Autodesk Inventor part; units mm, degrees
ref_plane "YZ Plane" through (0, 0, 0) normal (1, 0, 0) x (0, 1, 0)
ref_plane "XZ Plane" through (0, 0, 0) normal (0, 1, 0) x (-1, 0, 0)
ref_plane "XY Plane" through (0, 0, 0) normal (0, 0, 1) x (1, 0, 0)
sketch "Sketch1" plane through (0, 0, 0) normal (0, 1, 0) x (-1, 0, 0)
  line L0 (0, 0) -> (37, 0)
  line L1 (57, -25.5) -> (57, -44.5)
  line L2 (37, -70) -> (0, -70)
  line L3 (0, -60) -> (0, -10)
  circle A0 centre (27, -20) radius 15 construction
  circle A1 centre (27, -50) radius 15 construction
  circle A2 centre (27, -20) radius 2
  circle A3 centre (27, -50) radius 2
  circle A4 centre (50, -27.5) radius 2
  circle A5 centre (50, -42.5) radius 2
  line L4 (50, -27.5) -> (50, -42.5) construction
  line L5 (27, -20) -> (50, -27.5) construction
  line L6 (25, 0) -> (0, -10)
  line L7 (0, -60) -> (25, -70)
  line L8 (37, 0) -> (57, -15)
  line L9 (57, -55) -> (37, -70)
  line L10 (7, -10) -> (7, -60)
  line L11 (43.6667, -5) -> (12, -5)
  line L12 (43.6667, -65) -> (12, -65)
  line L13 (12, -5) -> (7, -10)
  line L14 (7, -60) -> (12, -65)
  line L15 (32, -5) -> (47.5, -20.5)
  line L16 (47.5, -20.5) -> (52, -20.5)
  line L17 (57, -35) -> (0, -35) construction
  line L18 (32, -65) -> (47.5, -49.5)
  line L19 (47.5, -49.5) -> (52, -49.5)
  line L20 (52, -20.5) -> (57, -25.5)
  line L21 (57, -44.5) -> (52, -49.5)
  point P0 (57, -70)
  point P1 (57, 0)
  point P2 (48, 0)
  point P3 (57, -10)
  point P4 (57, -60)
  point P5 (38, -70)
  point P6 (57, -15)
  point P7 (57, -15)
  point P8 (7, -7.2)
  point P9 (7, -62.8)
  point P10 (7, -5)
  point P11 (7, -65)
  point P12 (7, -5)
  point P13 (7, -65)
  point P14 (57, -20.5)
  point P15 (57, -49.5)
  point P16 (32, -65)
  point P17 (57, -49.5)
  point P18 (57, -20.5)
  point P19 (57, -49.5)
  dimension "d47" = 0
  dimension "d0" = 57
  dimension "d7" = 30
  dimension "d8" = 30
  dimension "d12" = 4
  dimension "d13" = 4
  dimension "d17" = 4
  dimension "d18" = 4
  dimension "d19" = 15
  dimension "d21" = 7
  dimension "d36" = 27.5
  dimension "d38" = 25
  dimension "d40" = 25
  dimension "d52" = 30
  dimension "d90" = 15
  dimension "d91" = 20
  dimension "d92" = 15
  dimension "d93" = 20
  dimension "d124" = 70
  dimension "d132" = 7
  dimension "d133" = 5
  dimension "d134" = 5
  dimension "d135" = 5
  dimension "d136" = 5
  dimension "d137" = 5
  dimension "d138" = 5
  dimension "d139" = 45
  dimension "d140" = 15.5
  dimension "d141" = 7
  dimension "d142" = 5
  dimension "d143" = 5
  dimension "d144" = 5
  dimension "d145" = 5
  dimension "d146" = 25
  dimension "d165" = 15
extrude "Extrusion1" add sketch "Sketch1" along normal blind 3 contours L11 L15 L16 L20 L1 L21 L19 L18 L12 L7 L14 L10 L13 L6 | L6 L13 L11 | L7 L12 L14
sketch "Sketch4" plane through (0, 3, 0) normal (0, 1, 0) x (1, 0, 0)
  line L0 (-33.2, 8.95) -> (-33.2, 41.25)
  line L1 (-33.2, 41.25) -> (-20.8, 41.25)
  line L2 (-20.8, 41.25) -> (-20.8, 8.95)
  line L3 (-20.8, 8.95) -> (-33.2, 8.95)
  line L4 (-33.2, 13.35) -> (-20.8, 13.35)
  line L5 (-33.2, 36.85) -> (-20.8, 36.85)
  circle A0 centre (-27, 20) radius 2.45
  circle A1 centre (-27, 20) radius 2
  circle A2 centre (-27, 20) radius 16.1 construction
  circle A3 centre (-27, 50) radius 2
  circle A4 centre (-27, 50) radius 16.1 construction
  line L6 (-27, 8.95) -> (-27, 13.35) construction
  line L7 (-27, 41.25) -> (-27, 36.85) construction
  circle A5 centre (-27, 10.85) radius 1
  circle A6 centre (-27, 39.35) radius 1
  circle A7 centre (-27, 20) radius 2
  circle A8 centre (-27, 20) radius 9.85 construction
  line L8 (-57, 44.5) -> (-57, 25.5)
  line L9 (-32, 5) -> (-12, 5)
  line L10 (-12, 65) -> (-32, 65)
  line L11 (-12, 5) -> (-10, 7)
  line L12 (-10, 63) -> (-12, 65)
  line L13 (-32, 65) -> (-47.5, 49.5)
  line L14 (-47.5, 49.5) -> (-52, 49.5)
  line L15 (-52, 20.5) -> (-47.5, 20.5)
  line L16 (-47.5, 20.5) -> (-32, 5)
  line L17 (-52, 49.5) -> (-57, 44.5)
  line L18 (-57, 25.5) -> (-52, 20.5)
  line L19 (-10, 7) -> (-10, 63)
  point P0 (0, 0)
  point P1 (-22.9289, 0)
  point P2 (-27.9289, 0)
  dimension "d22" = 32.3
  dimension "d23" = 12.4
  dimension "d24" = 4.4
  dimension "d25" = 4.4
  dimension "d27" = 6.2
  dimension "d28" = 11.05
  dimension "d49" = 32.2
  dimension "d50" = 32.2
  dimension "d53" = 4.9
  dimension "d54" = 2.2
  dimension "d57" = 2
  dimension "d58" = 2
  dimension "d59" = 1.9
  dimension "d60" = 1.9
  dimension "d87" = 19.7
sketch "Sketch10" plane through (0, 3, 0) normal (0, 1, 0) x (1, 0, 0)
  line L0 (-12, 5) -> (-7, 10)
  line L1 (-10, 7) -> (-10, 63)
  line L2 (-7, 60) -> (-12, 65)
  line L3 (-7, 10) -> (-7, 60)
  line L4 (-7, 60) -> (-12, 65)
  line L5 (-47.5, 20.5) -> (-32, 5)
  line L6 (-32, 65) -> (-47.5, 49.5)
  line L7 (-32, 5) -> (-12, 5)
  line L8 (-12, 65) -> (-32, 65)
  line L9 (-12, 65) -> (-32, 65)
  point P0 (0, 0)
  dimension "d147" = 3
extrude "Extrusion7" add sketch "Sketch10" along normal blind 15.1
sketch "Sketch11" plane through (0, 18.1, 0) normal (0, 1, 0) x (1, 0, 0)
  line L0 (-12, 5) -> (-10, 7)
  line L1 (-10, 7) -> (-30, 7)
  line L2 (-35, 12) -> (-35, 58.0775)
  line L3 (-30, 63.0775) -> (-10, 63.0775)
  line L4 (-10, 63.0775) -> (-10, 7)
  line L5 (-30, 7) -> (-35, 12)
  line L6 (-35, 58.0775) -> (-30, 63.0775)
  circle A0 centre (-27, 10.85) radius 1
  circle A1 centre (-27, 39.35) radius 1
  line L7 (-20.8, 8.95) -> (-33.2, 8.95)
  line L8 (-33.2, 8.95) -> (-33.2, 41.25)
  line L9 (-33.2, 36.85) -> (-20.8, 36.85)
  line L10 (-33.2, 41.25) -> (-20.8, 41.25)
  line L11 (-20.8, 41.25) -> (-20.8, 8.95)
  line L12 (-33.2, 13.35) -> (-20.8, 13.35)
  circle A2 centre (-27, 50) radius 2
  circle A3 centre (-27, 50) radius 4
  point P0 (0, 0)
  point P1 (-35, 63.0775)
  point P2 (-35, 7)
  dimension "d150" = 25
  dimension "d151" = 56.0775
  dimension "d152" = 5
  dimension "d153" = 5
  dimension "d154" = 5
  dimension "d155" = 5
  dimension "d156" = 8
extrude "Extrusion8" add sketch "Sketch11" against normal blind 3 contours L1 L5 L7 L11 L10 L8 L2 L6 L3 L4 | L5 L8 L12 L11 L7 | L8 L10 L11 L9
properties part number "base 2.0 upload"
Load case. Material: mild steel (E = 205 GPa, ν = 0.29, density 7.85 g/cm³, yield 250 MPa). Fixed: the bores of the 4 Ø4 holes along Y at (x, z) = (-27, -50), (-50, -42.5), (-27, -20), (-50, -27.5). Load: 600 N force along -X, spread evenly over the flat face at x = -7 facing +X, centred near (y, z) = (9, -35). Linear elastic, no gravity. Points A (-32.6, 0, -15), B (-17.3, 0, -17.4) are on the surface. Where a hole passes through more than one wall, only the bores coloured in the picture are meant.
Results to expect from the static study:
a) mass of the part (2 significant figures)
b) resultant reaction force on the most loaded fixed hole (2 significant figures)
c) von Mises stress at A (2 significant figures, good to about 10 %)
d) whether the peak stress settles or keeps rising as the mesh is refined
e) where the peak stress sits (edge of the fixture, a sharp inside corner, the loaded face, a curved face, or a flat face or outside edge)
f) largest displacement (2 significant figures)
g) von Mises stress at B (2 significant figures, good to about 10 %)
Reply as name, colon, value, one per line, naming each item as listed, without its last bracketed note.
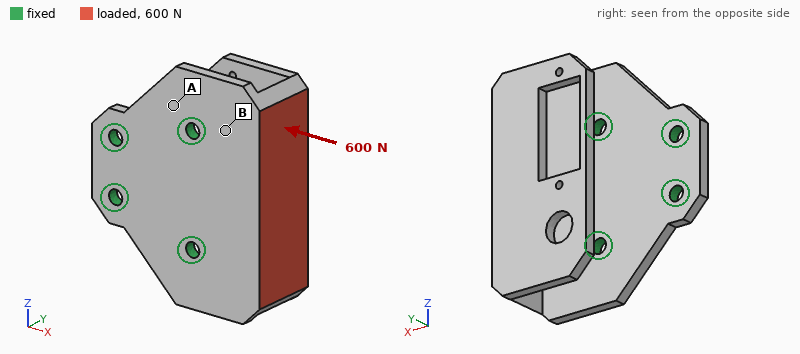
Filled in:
mass of the part: 99 g
resultant reaction force on the most loaded fixed hole: 250 N
von Mises stress at A: 8.3 MPa
whether the peak stress settles or keeps rising as the mesh is refined: keeps rising
where the peak stress sits: edge of the fixture
largest displacement: 93 µm
von Mises stress at B: 42 MPa
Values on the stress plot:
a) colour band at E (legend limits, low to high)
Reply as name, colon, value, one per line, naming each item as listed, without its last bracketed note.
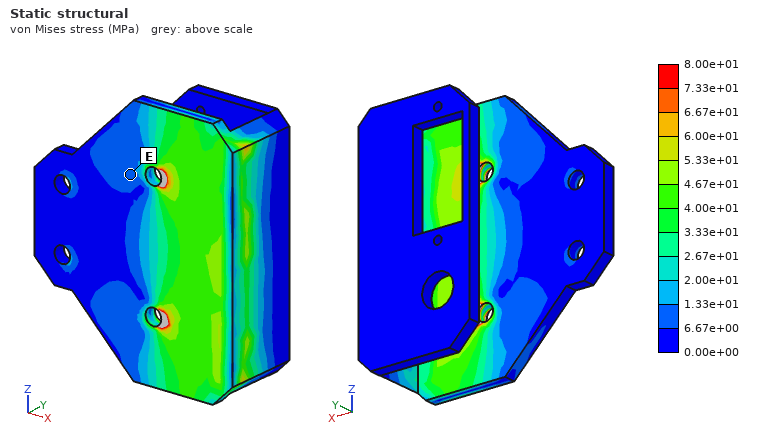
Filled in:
colour band at E: 6.67e+00 to 1.33e+01 MPa
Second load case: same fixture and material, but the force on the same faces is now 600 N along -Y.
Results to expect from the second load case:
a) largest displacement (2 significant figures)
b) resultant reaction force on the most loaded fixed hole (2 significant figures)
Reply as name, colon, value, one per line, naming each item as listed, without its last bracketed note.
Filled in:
largest displacement: 0.10 mm
resultant reaction force on the most loaded fixed hole: 370 N
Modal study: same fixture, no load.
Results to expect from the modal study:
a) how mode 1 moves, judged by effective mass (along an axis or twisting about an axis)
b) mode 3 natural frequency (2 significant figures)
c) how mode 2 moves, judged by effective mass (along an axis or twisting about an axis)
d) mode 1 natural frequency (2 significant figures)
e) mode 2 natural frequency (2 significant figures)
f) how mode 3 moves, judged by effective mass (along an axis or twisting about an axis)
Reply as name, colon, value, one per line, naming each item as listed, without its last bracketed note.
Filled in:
how mode 1 moves, judged by effective mass: along X
mode 3 natural frequency: 2700 Hz
how mode 2 moves, judged by effective mass: along Z
mode 1 natural frequency: 1600 Hz
mode 2 natural frequency: 2400 Hz
how mode 3 moves, judged by effective mass: along Y
